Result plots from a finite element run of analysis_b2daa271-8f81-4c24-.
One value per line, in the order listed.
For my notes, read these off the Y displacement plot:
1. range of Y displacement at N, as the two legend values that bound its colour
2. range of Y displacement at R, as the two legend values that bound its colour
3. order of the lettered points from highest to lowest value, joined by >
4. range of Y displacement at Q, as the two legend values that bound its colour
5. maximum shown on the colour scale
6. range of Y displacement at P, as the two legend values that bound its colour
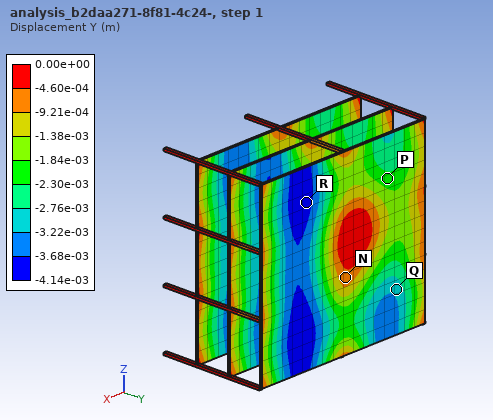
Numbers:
-9.21e-04 to -4.60e-04 m
-4.14e-03 to -3.68e-03 m
N > P > Q > R
-3.22e-03 to -2.76e-03 m
0.00e+00 m
-2.30e-03 to -1.84e-03 m
